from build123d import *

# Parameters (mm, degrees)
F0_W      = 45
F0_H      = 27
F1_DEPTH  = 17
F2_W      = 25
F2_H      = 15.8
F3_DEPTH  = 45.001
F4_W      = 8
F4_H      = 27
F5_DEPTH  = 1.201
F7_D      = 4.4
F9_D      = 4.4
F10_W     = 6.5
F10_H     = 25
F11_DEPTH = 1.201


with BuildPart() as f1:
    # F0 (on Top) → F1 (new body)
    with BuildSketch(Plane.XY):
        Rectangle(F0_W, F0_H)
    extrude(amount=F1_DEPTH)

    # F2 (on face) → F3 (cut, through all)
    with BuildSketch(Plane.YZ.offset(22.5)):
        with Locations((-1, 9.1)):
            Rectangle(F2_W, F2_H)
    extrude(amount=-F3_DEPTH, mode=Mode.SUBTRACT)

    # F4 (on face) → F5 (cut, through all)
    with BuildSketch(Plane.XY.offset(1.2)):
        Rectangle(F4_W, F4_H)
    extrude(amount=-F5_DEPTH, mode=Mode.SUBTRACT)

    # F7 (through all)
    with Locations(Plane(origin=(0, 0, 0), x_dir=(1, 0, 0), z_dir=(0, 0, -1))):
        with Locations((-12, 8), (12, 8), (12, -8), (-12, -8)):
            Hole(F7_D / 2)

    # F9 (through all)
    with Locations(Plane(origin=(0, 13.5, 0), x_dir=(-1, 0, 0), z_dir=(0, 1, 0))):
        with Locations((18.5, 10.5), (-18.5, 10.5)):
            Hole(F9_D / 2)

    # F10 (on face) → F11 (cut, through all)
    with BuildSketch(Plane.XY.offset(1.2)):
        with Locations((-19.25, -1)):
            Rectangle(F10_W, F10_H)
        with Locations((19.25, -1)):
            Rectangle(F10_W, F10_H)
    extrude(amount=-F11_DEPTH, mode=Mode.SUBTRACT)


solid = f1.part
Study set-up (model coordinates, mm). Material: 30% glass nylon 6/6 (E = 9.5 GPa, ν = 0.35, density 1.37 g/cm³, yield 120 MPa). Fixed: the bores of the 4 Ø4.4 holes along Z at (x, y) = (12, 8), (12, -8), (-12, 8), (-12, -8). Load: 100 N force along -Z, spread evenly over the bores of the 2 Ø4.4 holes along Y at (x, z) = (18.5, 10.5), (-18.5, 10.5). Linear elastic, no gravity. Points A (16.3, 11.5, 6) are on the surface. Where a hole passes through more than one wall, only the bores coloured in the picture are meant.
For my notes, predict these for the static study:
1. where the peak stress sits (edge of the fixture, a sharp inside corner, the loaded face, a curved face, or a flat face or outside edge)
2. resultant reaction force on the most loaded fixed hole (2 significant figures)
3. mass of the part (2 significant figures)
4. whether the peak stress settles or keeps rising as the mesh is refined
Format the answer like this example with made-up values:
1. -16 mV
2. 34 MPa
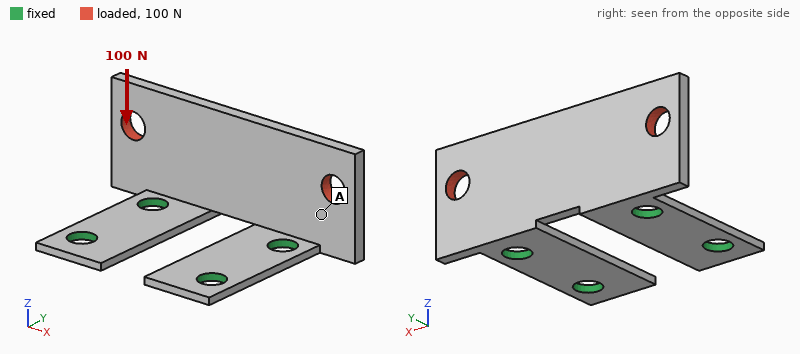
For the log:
1. edge of the fixture
2. 53 N
3. 2.9 g
4. keeps rising
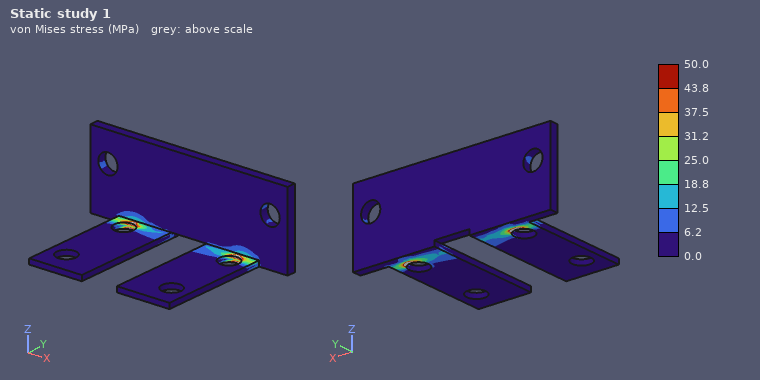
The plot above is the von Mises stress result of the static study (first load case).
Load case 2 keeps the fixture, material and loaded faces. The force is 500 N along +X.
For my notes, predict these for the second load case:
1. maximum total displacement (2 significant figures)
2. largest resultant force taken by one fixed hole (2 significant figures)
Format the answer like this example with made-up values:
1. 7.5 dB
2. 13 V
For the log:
1. 0.39 mm
2. 340 N
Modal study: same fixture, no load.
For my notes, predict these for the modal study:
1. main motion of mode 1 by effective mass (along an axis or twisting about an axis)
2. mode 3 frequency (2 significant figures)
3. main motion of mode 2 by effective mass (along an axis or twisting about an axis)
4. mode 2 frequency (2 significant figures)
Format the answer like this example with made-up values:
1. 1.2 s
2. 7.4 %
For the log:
1. along Y
2. 4800 Hz
3. twisting about Z
4. 2400 Hz
